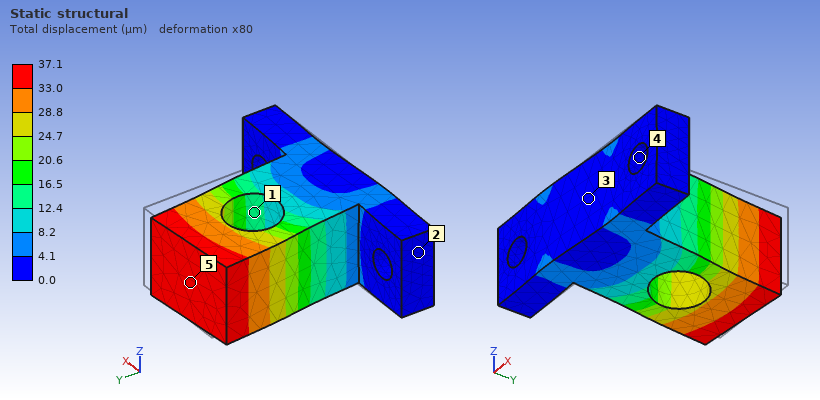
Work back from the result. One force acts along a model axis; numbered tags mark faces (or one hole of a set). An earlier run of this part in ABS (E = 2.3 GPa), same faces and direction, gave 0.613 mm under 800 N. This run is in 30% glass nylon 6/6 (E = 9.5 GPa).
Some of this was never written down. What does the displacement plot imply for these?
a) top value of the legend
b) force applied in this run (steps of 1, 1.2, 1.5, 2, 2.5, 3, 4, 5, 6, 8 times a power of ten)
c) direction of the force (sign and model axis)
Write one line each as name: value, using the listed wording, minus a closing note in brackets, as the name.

top value of the legend: 37.1 µm
force applied in this run: 200 N
direction of the force: -X
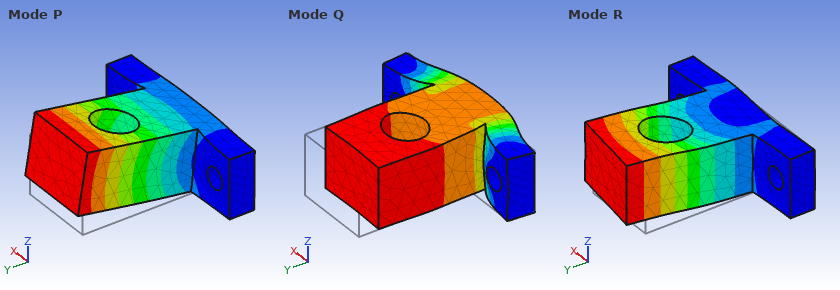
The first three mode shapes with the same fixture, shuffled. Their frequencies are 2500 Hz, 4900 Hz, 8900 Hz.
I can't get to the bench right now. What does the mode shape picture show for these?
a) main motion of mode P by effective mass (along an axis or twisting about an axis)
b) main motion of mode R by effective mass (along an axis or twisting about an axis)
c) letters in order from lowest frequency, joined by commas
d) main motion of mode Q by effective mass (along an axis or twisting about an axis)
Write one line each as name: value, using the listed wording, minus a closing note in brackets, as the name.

main motion of mode P by effective mass: along Z
main motion of mode R by effective mass: along X
letters in order from lowest frequency, joined by commas: P, R, Q
main motion of mode Q by effective mass: along Y
